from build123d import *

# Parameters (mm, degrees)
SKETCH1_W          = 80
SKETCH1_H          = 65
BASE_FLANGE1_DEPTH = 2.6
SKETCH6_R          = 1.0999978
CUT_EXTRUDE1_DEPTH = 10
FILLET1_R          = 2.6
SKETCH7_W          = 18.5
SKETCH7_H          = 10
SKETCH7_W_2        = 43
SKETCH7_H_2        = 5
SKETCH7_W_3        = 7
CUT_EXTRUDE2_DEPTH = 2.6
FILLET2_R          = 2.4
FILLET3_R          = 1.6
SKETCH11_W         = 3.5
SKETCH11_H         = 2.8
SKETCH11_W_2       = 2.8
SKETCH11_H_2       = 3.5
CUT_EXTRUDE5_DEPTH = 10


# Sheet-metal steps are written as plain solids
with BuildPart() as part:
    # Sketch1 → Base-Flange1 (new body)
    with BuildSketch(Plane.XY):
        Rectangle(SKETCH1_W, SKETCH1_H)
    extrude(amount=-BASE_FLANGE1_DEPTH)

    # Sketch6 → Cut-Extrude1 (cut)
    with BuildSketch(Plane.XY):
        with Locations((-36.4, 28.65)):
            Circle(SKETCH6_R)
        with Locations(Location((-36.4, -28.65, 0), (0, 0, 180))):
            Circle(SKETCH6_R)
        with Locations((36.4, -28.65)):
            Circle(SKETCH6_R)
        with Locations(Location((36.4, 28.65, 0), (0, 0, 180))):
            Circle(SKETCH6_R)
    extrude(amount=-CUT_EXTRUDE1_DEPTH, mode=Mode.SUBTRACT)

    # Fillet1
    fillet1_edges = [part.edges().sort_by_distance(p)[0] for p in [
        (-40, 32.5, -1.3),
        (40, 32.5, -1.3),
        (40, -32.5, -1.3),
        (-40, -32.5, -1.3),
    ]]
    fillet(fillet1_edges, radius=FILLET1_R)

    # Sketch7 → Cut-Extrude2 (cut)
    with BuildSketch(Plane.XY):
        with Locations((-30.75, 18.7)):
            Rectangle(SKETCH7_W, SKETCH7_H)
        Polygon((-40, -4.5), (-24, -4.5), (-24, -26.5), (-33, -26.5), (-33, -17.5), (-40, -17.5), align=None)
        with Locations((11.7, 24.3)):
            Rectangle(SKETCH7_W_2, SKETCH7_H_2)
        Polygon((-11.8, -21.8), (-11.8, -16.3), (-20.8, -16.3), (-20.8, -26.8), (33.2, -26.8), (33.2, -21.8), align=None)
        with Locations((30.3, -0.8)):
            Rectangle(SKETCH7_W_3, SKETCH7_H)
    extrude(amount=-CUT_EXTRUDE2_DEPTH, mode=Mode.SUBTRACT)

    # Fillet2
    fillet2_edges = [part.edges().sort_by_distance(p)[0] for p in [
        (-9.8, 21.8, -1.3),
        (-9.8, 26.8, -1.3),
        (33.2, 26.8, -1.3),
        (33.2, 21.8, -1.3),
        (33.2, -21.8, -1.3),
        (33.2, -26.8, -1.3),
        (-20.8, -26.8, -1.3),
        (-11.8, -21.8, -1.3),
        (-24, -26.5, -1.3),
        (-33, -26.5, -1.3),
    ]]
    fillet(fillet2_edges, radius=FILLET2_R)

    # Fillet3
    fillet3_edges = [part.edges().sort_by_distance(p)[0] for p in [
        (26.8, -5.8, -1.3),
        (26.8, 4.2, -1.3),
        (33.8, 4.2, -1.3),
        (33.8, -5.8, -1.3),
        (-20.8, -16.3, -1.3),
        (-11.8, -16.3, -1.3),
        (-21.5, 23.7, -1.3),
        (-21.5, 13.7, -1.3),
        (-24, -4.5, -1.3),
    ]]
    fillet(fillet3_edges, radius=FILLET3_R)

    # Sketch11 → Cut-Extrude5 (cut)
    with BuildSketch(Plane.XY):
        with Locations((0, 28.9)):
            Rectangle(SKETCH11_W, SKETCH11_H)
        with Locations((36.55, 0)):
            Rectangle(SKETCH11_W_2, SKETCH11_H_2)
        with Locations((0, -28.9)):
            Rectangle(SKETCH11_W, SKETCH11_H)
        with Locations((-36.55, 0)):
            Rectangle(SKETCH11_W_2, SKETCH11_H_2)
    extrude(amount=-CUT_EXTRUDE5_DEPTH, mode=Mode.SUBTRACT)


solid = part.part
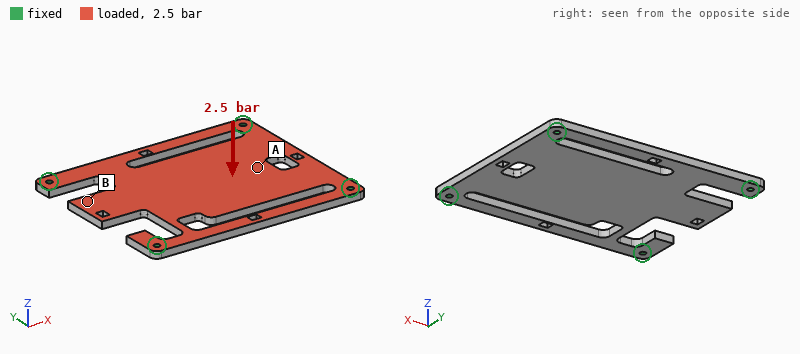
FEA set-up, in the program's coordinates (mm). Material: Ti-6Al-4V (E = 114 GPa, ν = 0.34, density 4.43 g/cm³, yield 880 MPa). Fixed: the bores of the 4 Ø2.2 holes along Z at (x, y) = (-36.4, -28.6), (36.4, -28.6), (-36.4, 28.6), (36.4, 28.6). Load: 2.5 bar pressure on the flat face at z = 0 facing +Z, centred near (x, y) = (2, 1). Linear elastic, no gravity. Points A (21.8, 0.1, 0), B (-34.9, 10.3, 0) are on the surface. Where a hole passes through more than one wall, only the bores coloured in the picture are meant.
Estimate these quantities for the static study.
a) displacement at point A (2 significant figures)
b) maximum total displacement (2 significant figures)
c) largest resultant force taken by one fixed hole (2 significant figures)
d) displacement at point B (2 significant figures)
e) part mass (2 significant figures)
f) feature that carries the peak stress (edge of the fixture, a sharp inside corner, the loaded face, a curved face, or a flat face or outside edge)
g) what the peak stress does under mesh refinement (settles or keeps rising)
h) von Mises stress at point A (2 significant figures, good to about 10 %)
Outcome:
0.21 mm
0.40 mm
270 N
0.33 mm
47 g
edge of the fixture
keeps rising
49 MPa
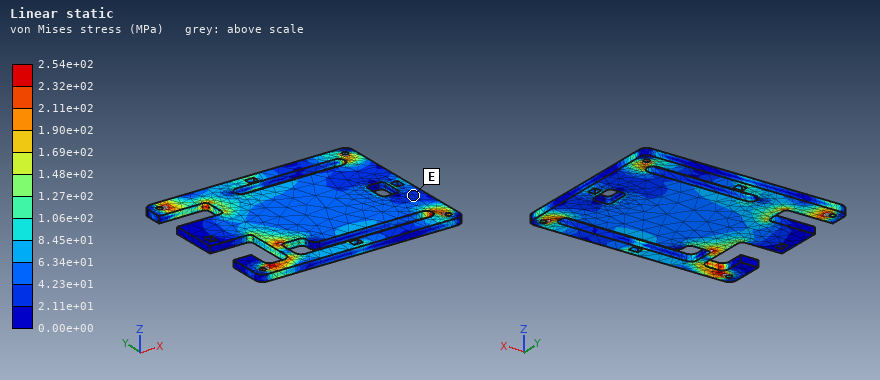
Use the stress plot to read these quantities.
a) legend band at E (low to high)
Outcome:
2.11e+01 to 4.23e+01 MPa
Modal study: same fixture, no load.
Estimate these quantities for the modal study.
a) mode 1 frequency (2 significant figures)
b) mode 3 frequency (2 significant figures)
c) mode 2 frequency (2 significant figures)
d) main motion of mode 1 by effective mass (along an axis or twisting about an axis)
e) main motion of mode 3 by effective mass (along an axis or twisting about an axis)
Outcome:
1400 Hz
2700 Hz
2200 Hz
along Z
twisting about X
